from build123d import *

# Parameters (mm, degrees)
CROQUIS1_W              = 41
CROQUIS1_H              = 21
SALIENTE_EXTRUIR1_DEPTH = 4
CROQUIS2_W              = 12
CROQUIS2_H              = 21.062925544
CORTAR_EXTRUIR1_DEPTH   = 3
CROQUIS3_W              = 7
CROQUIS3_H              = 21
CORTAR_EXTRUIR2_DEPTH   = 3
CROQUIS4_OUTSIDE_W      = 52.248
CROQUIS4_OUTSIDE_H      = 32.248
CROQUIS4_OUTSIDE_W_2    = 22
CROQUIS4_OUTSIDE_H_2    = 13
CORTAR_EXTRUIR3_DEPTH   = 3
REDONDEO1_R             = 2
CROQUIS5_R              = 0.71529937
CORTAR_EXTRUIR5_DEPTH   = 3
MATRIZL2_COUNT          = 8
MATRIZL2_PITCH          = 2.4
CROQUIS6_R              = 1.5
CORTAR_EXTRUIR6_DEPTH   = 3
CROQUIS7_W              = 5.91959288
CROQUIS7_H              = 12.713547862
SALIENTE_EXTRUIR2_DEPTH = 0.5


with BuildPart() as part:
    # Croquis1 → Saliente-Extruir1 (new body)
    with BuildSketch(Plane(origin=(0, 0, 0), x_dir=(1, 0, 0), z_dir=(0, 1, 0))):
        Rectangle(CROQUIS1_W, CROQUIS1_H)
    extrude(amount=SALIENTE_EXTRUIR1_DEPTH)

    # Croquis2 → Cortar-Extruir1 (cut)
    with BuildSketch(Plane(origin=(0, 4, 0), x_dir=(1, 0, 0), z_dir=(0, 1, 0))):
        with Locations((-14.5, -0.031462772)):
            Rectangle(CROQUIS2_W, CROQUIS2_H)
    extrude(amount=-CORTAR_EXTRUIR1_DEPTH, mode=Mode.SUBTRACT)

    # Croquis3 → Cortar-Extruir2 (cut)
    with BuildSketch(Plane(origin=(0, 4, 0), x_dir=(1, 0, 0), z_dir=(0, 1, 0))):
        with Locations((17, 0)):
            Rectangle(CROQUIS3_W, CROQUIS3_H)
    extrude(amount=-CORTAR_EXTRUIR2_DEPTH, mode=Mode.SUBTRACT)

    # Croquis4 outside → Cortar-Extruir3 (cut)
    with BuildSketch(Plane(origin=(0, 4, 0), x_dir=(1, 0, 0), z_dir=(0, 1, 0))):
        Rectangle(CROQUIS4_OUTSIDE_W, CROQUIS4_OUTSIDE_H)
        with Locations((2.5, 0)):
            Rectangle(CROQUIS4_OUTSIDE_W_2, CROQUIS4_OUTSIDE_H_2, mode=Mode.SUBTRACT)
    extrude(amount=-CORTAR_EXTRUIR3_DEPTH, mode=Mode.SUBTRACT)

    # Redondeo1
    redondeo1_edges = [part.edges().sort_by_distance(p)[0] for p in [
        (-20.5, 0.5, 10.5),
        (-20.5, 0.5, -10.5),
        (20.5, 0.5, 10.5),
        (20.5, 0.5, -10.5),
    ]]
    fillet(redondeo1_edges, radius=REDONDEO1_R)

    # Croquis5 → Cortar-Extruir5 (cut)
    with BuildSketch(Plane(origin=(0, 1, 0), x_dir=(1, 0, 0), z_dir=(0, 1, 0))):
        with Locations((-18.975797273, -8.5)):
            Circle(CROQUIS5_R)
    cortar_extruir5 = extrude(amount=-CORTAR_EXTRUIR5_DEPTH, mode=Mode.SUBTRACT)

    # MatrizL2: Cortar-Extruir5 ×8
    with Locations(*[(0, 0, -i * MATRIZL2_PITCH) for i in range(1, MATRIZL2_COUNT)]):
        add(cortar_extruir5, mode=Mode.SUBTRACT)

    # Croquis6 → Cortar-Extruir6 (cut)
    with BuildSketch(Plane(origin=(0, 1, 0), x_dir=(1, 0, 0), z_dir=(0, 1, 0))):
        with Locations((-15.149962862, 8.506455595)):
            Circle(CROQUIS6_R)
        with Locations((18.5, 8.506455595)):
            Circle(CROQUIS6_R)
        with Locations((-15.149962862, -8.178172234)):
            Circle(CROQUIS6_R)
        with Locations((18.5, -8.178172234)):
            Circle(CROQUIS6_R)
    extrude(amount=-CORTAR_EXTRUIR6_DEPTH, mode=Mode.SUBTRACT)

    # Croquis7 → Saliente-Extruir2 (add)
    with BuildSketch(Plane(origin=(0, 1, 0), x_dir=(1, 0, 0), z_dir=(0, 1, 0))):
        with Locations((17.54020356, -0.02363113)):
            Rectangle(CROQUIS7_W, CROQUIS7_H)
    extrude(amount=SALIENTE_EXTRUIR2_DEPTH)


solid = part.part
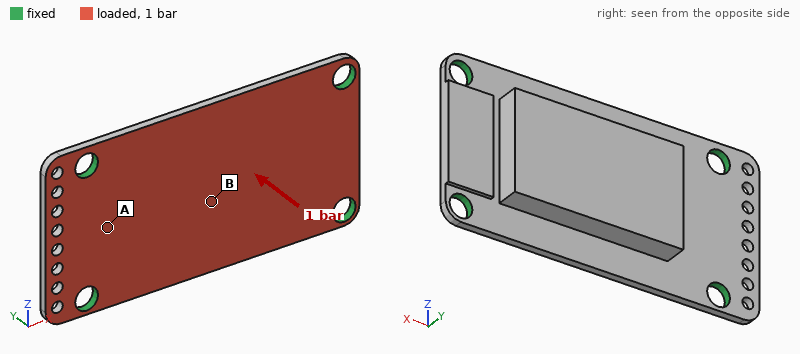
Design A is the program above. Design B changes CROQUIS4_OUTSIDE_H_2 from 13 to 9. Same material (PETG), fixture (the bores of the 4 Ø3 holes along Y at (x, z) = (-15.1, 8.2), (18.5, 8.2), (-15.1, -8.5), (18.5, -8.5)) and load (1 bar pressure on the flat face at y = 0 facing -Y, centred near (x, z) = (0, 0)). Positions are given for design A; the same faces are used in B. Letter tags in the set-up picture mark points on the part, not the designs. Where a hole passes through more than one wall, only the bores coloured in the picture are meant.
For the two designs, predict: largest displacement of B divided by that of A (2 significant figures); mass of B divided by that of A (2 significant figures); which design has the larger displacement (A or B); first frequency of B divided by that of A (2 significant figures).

1.5
0.85
B
0.96
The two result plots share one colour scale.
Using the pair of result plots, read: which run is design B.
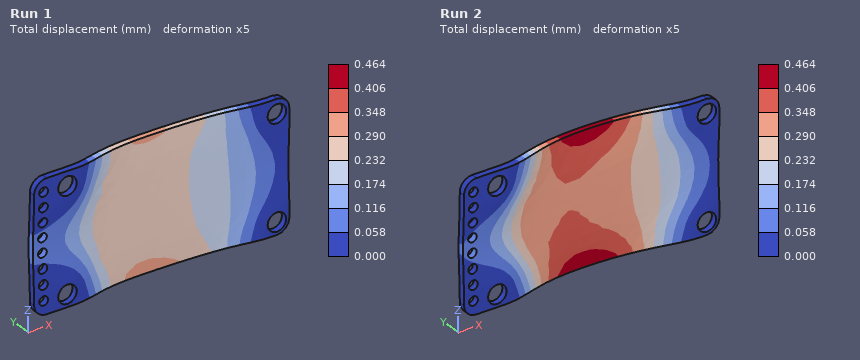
Run 2
